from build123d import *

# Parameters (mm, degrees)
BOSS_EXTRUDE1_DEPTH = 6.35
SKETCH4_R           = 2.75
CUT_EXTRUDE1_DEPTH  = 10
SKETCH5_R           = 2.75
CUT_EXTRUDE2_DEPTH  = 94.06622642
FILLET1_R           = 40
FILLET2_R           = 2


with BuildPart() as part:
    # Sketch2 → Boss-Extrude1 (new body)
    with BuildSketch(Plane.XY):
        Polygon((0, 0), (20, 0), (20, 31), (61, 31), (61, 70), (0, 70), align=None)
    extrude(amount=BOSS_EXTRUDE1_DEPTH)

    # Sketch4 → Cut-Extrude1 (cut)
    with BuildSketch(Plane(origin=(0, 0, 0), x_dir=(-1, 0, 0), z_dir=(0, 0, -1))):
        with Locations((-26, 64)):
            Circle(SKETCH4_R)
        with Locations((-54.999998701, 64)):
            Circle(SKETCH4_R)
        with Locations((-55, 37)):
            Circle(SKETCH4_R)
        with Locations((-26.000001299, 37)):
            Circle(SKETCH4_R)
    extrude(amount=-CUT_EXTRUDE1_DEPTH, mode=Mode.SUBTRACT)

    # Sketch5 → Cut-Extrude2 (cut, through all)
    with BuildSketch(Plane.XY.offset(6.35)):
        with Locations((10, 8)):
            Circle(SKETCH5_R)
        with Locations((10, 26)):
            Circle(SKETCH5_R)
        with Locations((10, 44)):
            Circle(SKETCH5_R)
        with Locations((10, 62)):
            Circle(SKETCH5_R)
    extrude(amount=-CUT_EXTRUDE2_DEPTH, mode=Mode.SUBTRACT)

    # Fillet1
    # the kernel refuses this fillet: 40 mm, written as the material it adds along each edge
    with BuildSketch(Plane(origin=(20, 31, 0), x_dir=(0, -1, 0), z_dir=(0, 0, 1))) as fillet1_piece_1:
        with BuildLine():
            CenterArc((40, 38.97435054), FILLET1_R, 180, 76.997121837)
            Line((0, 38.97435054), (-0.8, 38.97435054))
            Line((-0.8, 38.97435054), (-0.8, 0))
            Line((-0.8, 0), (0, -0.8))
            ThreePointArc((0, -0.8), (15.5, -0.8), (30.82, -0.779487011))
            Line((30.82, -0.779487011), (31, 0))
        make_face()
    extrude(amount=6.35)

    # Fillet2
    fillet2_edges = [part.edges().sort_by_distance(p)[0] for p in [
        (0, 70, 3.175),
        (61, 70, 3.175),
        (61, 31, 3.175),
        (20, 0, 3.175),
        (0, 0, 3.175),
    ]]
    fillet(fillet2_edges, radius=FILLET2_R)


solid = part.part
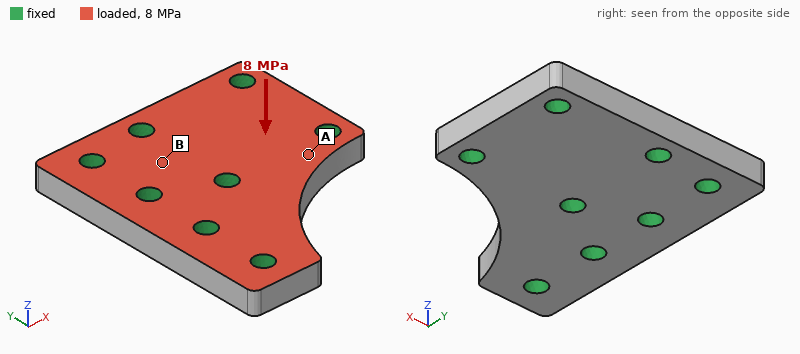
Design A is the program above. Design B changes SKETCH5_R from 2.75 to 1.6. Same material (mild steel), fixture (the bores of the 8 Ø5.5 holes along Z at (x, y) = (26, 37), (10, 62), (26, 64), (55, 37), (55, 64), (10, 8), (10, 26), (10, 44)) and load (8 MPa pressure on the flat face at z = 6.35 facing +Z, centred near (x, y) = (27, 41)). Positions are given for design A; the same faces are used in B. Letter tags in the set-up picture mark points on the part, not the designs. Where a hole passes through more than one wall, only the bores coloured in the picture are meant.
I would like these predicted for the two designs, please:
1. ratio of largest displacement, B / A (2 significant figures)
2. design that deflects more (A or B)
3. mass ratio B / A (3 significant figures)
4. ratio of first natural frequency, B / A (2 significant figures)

1.1
B
1.02
0.92
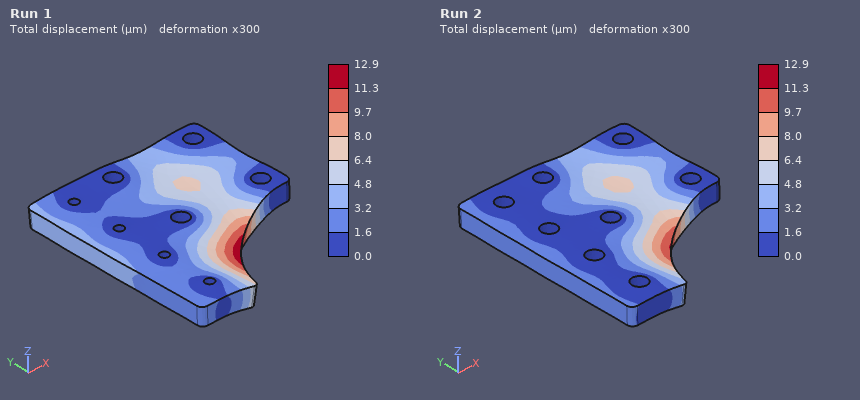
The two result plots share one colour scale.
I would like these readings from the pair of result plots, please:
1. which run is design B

Run 1
